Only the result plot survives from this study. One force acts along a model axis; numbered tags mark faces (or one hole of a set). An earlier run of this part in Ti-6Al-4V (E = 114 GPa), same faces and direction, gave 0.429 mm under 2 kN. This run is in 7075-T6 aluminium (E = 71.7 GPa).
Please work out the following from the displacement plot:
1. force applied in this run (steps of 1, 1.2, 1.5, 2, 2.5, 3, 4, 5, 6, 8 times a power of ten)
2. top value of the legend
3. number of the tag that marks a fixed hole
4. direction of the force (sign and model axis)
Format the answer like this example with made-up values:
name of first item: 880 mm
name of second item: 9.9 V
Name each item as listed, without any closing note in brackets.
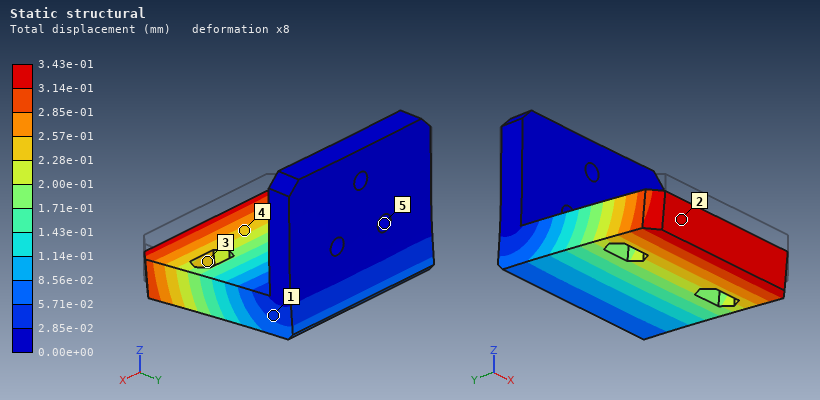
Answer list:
force applied in this run: 1 kN
top value of the legend: 3.43e-01 mm
number of the tag that marks a fixed hole: 5
direction of the force: -Z
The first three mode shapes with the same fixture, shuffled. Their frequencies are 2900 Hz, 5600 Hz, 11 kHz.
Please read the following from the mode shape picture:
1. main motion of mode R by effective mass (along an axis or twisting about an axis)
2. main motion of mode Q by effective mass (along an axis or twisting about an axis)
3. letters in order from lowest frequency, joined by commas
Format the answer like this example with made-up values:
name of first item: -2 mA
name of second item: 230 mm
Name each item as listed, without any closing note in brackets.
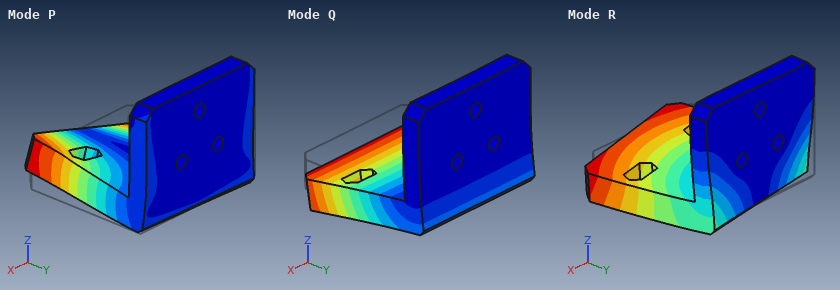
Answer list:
main motion of mode R by effective mass: along X
main motion of mode Q by effective mass: along Z
letters in order from lowest frequency, joined by commas: Q, R, P
